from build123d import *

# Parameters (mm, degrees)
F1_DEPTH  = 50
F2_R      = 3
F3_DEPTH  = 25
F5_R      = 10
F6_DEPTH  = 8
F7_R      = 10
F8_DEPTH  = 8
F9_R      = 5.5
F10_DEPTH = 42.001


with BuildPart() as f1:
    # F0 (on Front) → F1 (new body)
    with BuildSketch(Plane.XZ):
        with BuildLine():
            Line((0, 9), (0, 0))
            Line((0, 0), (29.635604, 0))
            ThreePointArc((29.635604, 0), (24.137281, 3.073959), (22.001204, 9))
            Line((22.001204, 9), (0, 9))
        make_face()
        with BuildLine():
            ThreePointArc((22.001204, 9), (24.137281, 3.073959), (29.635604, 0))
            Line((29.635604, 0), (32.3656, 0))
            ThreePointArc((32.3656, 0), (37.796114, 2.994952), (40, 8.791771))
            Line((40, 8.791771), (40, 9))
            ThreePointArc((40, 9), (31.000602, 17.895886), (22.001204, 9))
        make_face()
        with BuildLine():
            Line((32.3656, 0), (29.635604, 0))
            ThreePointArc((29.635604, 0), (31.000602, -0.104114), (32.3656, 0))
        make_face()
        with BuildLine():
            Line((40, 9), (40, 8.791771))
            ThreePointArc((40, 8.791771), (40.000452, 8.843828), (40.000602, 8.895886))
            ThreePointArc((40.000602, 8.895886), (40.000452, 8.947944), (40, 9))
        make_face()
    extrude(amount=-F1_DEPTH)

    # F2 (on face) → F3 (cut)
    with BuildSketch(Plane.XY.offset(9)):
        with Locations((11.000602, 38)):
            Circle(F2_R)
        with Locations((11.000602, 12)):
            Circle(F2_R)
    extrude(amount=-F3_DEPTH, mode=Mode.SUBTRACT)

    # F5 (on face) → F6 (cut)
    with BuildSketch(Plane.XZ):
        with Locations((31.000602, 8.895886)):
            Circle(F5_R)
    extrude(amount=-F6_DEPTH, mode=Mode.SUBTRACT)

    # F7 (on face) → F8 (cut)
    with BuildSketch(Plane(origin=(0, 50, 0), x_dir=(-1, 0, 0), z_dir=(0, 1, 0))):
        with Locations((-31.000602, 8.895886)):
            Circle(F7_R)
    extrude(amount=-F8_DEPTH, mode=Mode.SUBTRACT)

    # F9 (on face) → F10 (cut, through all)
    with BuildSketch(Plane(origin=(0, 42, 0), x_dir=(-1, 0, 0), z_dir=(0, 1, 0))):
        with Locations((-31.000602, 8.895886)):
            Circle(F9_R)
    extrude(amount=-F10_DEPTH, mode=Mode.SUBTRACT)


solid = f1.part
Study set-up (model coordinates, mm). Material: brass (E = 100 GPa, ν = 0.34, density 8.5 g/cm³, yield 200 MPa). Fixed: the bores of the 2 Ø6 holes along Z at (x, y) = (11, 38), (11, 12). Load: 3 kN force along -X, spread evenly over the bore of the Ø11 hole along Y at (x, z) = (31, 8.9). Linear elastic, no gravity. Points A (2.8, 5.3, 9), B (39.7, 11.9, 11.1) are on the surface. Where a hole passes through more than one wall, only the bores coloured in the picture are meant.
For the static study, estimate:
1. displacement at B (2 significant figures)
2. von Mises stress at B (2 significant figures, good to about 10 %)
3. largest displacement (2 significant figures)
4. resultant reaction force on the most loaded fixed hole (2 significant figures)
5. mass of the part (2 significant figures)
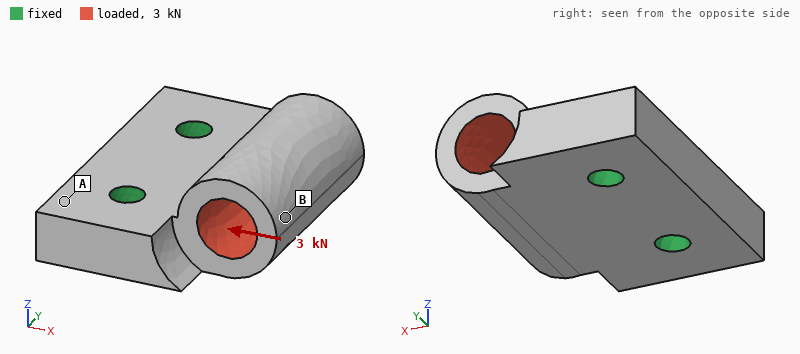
29 µm
17 MPa
29 µm
1.5 kN
130 g
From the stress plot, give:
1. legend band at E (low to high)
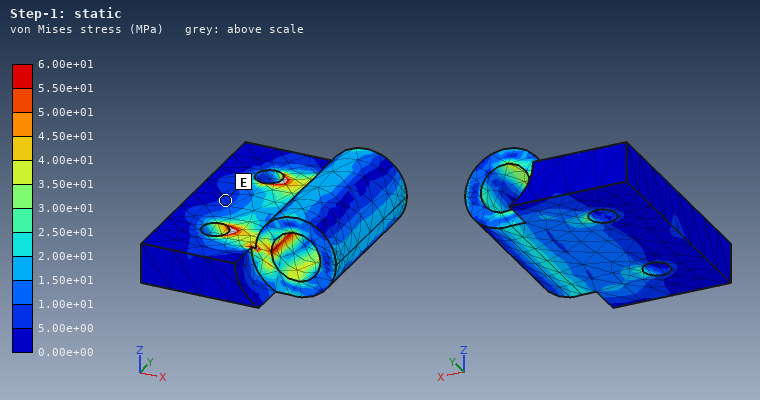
5.00e+00 to 1.00e+01 MPa
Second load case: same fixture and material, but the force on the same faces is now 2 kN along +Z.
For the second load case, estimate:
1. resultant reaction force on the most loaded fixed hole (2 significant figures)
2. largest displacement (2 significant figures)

1.0 kN
50 µm
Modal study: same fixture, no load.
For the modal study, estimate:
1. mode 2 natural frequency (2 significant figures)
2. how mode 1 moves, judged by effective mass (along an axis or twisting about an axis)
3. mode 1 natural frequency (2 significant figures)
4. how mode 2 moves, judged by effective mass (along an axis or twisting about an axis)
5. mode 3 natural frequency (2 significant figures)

12 kHz
along Z
5000 Hz
along Y
14 kHz
